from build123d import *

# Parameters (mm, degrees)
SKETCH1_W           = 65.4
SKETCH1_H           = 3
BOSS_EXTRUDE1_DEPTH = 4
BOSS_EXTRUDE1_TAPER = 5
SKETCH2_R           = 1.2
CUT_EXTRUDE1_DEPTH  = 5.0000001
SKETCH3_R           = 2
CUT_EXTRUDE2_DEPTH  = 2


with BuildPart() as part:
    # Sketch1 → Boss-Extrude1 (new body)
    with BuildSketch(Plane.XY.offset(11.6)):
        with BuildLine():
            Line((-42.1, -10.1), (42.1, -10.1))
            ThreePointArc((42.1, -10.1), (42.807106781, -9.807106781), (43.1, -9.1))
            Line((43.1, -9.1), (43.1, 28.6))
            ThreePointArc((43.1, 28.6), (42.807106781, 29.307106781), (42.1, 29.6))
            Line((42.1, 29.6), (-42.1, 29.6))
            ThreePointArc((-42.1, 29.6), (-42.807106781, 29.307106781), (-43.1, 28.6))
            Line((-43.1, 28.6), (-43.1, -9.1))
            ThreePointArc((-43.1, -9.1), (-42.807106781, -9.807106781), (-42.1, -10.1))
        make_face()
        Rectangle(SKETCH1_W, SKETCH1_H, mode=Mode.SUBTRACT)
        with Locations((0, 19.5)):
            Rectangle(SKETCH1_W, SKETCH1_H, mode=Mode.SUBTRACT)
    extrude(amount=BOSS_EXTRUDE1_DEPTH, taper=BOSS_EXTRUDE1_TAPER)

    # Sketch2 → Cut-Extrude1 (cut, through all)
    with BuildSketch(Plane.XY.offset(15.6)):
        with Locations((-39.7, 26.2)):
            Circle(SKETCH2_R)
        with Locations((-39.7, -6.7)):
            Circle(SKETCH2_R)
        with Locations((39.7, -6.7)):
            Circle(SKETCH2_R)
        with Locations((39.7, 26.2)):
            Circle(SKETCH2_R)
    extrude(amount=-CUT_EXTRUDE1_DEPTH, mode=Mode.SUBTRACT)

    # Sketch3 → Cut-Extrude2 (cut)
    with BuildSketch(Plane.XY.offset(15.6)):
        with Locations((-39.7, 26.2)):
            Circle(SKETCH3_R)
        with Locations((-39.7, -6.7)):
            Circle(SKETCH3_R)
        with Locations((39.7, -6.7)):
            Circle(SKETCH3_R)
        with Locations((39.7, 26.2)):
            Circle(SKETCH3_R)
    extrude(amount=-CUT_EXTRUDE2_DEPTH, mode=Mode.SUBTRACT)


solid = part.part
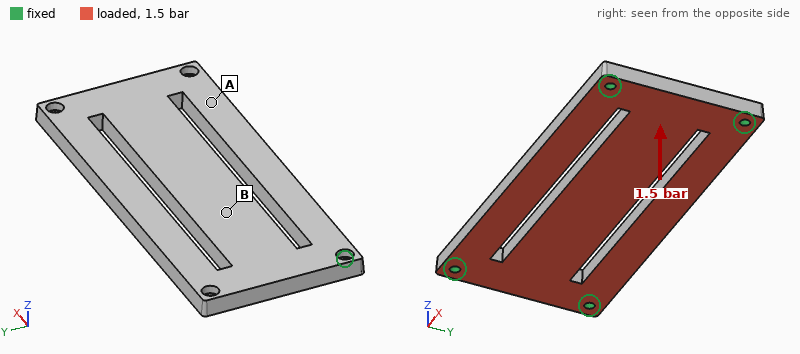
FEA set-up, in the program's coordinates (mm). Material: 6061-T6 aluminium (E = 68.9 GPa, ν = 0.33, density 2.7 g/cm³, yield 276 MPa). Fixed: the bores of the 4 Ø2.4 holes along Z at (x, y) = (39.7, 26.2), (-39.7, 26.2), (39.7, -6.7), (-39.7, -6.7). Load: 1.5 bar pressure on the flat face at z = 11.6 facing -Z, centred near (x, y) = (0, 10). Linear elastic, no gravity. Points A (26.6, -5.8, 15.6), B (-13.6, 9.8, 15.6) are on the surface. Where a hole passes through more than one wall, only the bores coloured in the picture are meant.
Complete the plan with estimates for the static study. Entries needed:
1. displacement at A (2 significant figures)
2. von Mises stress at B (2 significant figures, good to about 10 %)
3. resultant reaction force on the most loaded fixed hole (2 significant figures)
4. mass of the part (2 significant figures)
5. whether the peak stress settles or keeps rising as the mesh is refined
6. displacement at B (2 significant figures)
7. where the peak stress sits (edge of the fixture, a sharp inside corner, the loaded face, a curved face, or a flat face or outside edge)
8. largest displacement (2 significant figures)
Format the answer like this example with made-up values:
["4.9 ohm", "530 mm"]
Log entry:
["32 µm", "19 MPa", "190 N", "31 g", "keeps rising", "78 µm", "edge of the fixture", "95 µm"]
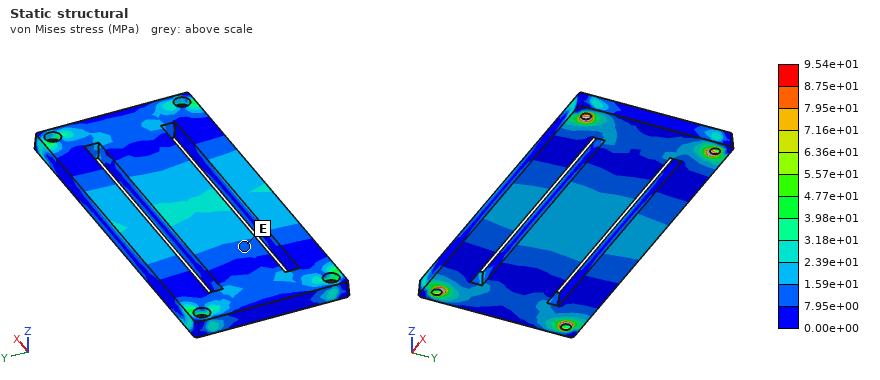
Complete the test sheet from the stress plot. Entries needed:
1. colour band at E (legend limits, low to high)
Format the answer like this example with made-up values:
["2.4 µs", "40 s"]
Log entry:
["7.95e+00 to 1.59e+01 MPa"]
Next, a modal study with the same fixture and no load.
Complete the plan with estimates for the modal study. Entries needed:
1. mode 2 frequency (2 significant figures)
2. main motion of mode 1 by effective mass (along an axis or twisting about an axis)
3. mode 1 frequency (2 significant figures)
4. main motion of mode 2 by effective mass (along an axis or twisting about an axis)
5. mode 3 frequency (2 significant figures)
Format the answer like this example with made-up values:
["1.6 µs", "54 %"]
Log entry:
["3100 Hz", "along Z", "2300 Hz", "twisting about X", "3400 Hz"]
